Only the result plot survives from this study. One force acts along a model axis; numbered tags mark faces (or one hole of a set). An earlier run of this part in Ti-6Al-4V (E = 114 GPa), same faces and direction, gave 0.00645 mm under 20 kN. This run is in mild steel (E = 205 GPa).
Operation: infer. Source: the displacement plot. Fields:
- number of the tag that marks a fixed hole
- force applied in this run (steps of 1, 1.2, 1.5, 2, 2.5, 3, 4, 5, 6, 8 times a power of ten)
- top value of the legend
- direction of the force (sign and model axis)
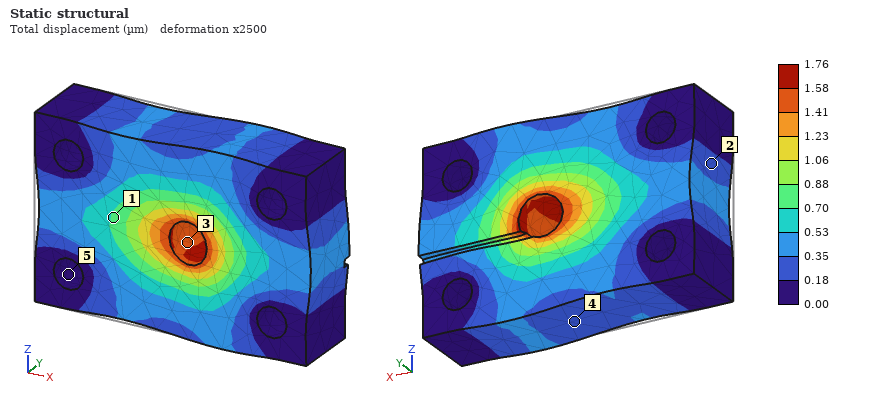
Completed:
5
10 kN
1.76 µm
+X
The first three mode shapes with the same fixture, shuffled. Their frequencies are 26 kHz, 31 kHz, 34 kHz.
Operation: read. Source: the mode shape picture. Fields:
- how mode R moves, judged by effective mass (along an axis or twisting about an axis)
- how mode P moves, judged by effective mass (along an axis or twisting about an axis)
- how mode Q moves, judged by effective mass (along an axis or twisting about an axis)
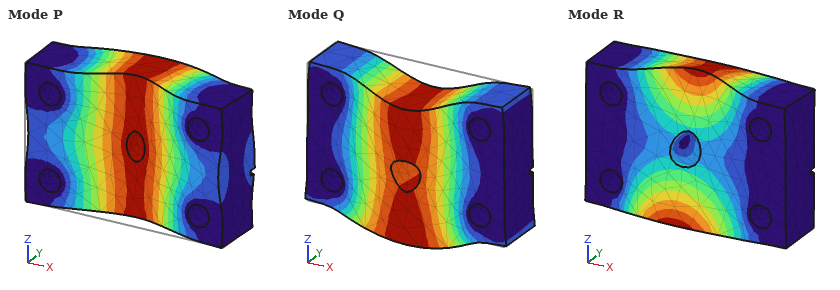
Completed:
twisting about X
along Y
along Z
